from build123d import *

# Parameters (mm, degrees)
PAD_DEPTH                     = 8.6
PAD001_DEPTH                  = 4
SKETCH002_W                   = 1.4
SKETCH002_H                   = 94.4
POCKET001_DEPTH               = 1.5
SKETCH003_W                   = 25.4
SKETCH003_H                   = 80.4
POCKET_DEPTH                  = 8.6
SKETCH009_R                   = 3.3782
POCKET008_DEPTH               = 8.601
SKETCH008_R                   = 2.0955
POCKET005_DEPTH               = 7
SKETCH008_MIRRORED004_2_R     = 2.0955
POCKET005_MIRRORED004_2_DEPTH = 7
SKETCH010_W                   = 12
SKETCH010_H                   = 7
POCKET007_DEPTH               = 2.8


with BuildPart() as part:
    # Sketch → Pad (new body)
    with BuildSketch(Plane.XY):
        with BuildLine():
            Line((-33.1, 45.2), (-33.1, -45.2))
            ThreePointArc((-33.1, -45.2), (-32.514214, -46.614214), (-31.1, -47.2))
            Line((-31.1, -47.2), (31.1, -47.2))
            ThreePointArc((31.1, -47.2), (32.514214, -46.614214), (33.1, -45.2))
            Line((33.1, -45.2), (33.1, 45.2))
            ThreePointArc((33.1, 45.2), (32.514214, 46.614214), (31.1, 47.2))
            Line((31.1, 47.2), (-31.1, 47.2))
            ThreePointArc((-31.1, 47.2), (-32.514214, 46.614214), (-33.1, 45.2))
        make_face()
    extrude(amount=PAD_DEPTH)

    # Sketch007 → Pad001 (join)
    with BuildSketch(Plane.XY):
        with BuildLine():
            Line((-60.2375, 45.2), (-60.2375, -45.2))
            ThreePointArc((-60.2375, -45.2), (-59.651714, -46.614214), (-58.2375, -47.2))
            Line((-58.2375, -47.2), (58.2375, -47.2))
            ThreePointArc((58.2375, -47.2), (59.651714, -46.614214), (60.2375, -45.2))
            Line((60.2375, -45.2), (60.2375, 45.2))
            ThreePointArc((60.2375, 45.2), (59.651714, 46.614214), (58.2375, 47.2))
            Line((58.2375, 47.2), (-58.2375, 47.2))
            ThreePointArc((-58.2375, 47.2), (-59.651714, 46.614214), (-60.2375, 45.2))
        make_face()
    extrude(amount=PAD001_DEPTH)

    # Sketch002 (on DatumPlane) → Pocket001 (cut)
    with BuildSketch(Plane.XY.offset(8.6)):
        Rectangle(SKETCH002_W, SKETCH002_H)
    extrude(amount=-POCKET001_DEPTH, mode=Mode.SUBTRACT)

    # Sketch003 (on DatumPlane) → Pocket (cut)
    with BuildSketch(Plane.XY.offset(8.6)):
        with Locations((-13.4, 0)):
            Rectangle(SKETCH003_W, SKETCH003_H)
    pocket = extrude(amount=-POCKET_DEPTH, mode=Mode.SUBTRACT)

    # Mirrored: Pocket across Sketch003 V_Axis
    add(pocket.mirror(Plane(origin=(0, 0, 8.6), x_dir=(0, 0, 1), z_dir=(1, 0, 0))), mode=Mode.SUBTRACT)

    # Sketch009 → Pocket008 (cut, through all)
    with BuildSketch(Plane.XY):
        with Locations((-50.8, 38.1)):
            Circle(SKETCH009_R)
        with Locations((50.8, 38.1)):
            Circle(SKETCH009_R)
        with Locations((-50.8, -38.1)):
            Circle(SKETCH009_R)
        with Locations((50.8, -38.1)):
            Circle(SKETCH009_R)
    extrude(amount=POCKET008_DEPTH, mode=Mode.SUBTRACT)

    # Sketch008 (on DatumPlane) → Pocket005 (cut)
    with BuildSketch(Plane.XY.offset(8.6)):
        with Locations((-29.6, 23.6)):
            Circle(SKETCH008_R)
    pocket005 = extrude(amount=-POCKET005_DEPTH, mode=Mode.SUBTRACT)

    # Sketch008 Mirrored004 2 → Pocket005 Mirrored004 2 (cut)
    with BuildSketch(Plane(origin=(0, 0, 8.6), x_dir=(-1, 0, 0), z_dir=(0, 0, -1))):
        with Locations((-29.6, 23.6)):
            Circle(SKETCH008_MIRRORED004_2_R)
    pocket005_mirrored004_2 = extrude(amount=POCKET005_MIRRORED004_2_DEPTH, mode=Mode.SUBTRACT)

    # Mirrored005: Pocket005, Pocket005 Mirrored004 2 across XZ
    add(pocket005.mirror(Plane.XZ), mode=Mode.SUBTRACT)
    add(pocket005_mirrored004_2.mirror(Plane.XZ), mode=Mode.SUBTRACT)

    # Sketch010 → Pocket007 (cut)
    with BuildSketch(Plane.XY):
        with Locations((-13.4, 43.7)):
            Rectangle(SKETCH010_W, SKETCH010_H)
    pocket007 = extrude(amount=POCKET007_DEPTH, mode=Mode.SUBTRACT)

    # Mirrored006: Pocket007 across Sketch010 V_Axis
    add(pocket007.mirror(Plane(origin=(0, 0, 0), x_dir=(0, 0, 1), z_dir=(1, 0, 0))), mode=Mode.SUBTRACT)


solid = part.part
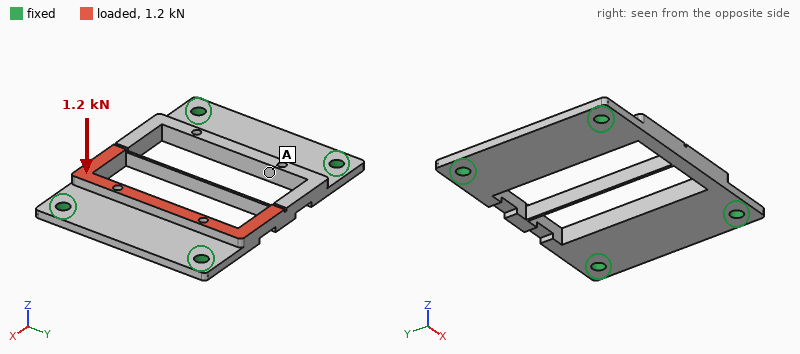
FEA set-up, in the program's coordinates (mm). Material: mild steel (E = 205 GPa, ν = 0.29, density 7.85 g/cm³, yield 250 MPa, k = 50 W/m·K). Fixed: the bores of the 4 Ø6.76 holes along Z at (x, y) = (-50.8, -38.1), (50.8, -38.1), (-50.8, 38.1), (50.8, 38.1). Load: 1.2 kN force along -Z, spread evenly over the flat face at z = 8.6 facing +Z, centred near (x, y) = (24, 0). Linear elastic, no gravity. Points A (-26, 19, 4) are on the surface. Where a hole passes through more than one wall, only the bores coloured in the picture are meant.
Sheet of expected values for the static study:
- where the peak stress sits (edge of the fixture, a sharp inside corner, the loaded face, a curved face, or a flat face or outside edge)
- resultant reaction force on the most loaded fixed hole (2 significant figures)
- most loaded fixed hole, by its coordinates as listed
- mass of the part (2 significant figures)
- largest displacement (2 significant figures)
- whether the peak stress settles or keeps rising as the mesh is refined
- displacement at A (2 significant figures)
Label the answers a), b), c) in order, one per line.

a) edge of the fixture
b) 740 N
c) (50.8, 38.1)
d) 290 g
e) 44 µm
f) keeps rising
g) 10 µm
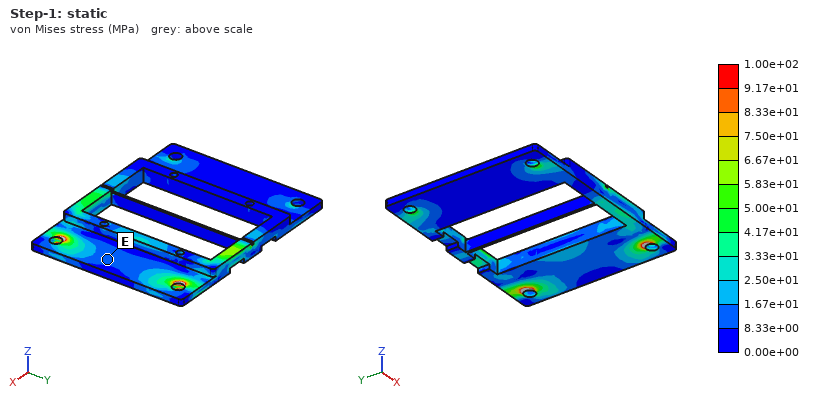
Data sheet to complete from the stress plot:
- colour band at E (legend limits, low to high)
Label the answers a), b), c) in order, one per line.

a) 8.33e+00 to 1.67e+01 MPa
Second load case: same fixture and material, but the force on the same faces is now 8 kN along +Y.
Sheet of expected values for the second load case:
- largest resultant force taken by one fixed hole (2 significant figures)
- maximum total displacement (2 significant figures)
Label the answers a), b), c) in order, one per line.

a) 4.2 kN
b) 63 µm
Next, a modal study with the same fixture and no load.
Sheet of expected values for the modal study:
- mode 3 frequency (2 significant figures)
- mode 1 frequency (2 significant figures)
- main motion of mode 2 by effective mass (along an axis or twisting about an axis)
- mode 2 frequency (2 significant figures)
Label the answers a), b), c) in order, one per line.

a) 3100 Hz
b) 1100 Hz
c) along Z
d) 2700 Hz
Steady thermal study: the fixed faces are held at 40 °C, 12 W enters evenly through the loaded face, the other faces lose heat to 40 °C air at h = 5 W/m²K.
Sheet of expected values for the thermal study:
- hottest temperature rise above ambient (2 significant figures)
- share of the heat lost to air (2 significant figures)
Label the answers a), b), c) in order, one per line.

a) 20 K
b) 6.5 %
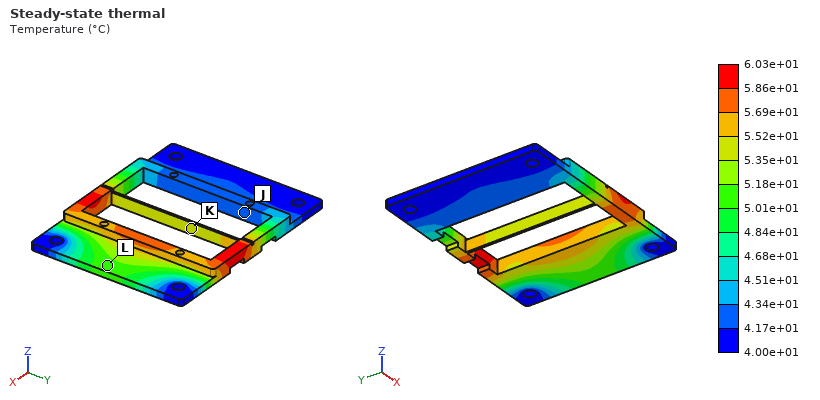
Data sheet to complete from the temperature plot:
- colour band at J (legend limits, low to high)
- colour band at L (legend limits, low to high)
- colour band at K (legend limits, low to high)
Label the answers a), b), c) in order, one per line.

a) 4.17e+01 to 4.34e+01 °C
b) 5.01e+01 to 5.18e+01 °C
c) 5.35e+01 to 5.52e+01 °C
